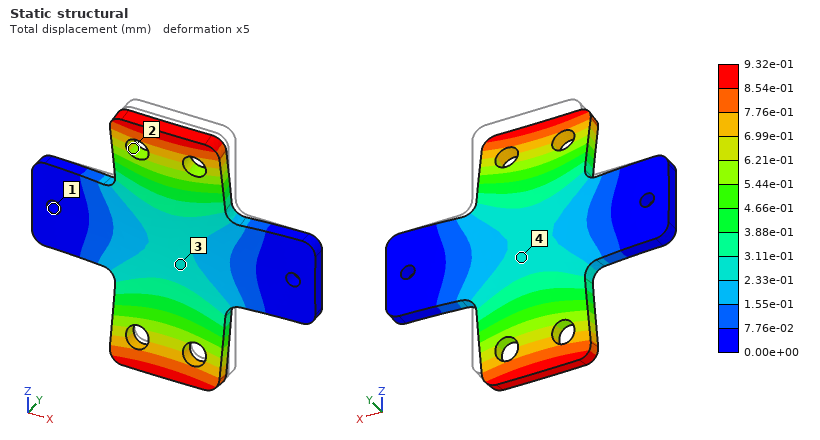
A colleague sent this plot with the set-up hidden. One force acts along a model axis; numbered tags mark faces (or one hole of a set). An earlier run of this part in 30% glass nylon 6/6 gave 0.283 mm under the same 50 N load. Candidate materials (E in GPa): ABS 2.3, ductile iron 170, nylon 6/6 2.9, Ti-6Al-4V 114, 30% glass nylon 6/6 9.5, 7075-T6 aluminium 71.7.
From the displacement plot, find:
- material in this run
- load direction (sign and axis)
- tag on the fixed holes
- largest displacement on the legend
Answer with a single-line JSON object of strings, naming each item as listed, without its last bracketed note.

{"material in this run": "nylon 6/6", "load direction": "-Y", "tag on the fixed holes": "1", "largest displacement on the legend": "9.32e-01 mm"}
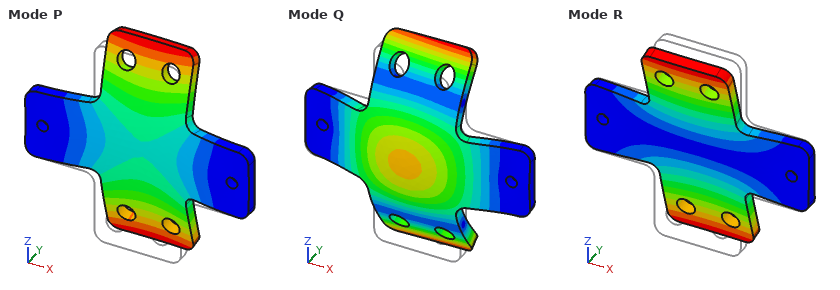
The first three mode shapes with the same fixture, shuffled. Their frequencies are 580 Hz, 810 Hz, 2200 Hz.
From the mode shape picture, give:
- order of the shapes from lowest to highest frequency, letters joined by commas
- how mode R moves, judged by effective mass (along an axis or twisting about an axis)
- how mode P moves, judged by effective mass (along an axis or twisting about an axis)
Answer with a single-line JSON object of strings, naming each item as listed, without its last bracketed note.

{"order of the shapes from lowest to highest frequency, letters joined by commas": "R, P, Q", "how mode R moves, judged by effective mass": "twisting about X", "how mode P moves, judged by effective mass": "along Y"}
